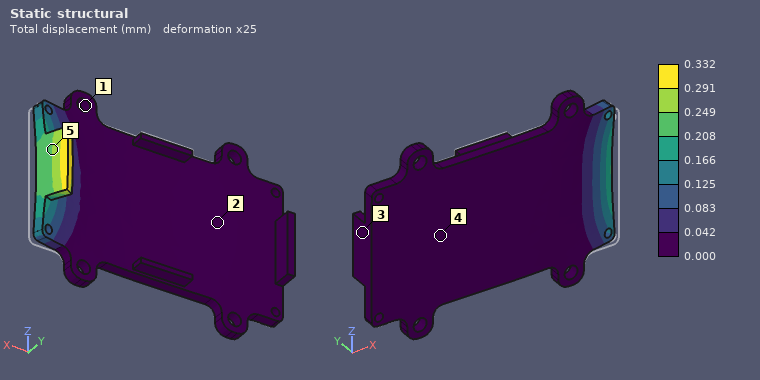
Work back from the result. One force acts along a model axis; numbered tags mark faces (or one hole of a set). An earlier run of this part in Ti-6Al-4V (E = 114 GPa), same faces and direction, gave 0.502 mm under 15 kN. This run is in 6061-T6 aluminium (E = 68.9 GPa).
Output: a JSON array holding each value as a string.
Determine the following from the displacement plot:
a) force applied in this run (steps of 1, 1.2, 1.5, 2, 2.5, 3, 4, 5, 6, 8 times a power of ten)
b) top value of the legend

["6 kN", "0.332 mm"]
